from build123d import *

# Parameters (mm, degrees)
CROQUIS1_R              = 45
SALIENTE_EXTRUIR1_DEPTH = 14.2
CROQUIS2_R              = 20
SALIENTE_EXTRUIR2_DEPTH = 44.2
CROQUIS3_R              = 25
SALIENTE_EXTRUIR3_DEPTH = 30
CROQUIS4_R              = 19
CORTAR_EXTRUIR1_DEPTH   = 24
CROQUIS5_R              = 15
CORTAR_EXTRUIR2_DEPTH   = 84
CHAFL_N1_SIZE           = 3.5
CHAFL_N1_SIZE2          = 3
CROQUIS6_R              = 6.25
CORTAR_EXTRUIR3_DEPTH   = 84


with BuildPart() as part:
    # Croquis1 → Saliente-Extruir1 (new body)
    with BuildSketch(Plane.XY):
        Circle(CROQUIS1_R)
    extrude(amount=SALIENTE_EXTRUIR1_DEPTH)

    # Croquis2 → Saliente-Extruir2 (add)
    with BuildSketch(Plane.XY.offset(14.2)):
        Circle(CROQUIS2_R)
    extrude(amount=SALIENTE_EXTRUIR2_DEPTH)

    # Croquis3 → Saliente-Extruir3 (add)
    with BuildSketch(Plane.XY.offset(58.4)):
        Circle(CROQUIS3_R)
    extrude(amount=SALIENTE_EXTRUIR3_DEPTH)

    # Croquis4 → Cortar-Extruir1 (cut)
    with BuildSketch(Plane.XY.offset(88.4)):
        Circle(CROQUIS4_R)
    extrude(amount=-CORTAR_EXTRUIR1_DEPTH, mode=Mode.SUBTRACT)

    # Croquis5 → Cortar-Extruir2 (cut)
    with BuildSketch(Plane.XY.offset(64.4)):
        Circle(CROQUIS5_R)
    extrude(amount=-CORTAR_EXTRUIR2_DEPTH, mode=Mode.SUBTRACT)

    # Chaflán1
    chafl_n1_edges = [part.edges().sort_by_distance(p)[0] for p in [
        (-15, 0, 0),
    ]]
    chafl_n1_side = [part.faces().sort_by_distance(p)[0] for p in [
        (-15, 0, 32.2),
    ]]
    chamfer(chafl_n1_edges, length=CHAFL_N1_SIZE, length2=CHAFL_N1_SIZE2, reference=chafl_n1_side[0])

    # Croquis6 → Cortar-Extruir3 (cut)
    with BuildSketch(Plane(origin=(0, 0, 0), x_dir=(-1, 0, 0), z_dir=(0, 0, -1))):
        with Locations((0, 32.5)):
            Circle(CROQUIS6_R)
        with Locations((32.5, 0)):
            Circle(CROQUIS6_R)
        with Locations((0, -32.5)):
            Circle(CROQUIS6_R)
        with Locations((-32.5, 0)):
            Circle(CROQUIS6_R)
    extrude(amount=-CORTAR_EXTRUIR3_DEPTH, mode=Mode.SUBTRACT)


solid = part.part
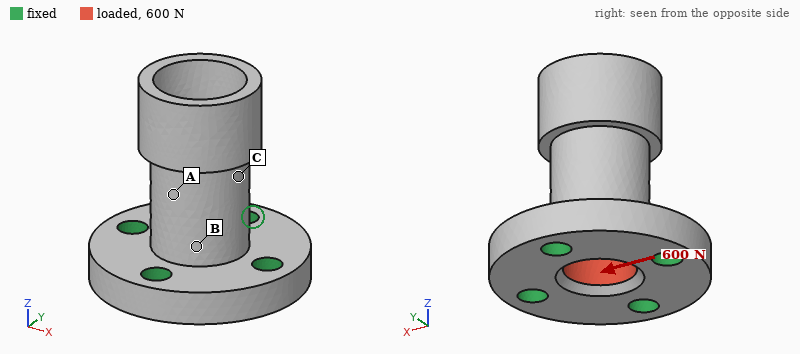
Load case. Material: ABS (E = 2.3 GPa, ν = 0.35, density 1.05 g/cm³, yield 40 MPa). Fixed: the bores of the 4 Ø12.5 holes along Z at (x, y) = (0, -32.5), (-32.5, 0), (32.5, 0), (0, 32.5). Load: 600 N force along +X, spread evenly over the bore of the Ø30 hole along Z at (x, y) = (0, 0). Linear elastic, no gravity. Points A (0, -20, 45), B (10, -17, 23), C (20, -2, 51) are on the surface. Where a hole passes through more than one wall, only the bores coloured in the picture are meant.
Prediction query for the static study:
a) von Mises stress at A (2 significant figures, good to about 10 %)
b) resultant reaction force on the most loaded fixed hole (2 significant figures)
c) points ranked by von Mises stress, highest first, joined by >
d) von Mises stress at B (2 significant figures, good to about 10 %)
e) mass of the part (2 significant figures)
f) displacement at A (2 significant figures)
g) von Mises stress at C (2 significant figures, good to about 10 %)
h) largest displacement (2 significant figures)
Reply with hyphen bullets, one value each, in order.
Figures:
- 1.1 MPa
- 340 N
- B > A > C
- 1.7 MPa
- 130 g
- 0.088 mm
- 0.40 MPa
- 0.18 mm
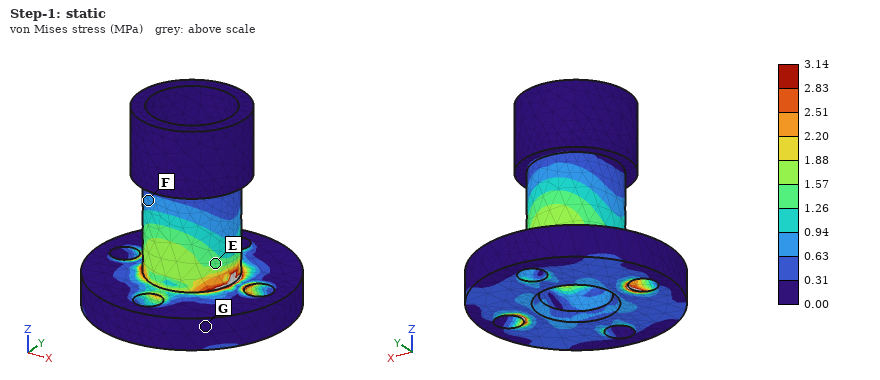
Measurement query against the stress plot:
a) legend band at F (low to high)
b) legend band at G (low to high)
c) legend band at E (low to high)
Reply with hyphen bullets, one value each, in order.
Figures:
- 0.63 to 0.94 MPa
- 0.00 to 0.31 MPa
- 1.26 to 1.57 MPa
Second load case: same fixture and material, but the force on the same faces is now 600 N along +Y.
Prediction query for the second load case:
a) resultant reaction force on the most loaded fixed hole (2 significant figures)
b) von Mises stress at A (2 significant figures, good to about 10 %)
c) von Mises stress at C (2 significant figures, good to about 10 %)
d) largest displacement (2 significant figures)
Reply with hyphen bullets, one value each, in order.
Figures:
- 340 N
- 0.56 MPa
- 0.78 MPa
- 0.18 mm
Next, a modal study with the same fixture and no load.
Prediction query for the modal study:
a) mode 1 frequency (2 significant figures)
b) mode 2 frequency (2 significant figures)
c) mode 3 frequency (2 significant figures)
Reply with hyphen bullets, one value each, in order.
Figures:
- 950 Hz
- 950 Hz
- 2100 Hz
